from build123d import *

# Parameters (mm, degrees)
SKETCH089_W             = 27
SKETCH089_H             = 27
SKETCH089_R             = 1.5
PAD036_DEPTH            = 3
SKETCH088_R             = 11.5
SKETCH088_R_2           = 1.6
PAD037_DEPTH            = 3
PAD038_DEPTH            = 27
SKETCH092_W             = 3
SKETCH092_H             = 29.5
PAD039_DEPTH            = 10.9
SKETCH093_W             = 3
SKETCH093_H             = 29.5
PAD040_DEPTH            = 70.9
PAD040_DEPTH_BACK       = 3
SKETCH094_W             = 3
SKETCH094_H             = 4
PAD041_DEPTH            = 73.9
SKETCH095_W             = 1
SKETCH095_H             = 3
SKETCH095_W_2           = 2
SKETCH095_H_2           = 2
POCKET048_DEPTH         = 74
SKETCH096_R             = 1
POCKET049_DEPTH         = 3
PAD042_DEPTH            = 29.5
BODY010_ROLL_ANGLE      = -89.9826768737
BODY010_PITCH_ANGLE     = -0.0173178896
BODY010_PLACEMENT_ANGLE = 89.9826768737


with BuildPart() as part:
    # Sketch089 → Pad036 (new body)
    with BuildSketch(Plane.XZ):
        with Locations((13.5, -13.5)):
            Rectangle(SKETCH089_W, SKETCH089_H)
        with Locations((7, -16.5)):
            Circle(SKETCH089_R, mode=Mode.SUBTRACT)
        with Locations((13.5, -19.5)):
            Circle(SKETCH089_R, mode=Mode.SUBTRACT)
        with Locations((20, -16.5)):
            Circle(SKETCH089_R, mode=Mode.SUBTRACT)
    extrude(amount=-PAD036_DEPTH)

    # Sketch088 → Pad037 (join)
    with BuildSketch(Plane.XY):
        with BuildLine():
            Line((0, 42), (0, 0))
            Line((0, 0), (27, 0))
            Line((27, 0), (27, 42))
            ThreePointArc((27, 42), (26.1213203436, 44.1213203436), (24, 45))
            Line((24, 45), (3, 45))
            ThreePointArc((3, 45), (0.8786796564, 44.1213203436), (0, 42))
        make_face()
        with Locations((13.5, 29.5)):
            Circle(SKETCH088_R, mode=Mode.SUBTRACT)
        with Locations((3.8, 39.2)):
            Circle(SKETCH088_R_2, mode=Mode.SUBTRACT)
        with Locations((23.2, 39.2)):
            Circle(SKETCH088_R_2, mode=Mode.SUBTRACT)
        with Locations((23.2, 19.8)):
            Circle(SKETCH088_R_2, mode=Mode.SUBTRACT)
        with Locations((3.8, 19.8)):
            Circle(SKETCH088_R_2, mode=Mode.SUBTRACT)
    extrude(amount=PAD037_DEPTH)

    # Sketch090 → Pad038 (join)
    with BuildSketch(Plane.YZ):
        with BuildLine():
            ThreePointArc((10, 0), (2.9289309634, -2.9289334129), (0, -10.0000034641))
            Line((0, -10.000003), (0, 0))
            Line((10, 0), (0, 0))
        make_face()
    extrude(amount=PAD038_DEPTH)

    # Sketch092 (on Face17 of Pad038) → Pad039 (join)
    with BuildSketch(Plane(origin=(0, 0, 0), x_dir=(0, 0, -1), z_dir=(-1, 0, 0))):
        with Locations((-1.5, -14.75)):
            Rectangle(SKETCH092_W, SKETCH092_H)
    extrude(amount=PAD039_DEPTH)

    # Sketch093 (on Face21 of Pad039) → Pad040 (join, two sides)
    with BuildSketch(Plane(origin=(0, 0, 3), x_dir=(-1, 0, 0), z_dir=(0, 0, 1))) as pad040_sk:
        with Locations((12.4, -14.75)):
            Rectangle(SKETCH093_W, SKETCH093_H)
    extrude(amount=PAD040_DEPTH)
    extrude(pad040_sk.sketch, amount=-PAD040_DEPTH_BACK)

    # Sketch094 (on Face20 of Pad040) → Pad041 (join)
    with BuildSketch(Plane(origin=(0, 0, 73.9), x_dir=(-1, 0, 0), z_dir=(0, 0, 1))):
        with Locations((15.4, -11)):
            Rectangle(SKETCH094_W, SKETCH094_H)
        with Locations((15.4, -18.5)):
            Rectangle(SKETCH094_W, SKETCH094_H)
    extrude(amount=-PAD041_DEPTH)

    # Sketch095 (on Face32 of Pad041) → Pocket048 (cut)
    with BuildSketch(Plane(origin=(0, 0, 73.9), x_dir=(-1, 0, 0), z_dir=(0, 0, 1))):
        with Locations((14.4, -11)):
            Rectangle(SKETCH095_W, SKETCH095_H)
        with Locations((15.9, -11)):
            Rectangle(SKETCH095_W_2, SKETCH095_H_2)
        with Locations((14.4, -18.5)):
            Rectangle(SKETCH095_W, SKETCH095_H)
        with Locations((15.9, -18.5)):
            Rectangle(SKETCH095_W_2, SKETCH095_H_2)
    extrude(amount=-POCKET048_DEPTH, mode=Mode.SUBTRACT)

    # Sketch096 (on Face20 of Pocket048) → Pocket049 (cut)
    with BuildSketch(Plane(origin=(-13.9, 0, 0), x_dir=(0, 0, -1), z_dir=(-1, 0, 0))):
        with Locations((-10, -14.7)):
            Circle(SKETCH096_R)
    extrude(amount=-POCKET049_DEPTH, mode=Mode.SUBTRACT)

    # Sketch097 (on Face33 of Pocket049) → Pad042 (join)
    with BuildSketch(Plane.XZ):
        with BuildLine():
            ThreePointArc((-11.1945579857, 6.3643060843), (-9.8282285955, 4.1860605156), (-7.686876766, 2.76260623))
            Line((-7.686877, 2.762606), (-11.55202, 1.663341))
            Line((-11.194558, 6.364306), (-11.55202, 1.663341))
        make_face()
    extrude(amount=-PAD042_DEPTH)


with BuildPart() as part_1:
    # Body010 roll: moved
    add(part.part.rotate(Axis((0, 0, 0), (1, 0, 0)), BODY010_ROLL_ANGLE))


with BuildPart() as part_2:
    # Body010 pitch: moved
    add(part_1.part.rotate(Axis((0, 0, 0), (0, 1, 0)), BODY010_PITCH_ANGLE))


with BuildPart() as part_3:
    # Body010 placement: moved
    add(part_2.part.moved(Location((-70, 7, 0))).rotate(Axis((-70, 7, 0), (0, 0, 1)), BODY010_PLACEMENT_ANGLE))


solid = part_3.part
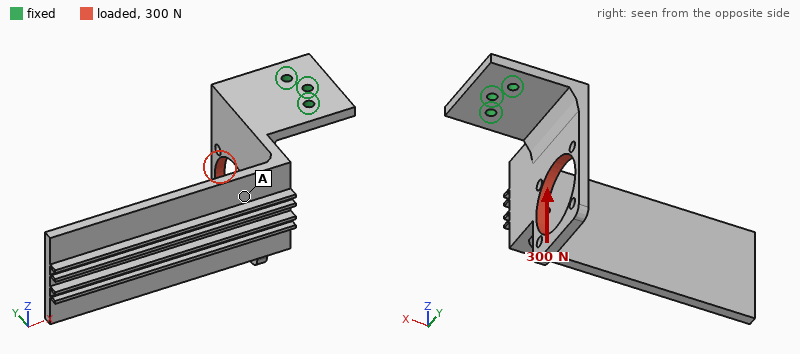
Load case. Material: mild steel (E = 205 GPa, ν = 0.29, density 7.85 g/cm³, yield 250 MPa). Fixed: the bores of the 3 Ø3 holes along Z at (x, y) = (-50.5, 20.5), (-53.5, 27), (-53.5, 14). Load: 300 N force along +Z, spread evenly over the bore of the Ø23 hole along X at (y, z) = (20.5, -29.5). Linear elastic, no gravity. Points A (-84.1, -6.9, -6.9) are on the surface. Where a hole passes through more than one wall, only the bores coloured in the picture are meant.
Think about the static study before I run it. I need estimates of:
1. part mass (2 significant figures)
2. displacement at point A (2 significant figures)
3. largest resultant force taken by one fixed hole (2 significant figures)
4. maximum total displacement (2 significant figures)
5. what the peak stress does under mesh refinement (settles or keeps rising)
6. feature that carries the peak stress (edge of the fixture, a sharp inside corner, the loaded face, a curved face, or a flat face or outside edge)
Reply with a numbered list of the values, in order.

1. 100 g
2. 0.092 mm
3. 210 N
4. 0.32 mm
5. keeps rising
6. edge of the fixture
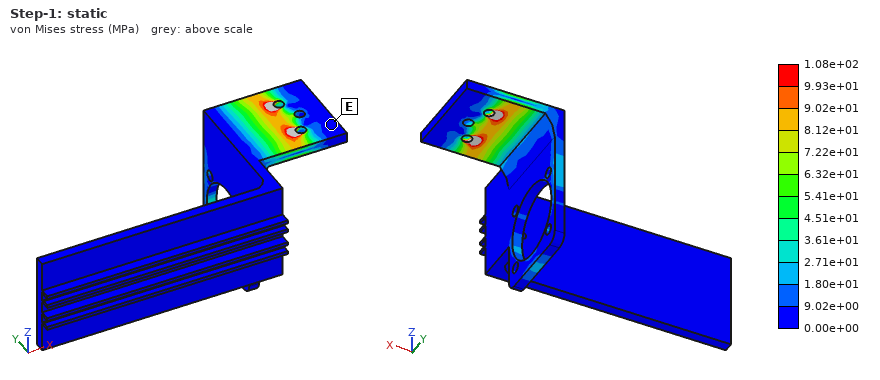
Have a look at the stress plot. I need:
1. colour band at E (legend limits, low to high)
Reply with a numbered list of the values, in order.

1. 0.00e+00 to 9.02e+00 MPa
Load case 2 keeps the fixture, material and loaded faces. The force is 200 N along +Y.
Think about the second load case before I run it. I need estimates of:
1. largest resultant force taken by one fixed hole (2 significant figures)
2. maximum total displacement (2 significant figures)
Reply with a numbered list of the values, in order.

1. 420 N
2. 0.11 mm
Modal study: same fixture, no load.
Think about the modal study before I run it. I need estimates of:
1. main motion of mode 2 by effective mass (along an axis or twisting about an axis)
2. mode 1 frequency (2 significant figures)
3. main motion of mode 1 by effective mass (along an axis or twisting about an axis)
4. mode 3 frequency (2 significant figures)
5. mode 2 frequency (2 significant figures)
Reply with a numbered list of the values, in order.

1. along Y
2. 270 Hz
3. along Z
4. 1400 Hz
5. 370 Hz
